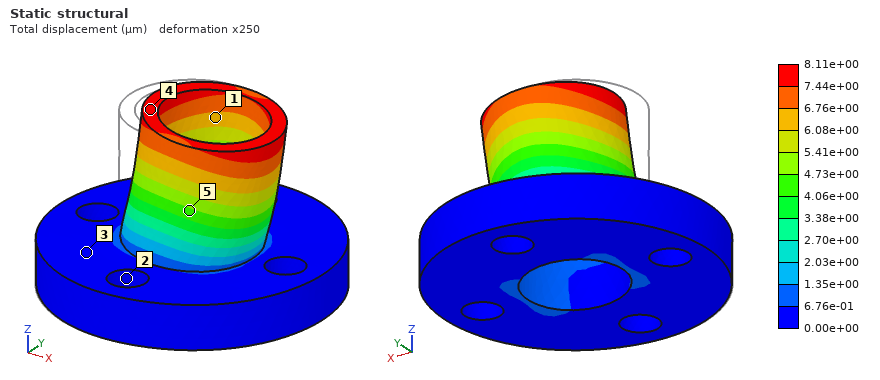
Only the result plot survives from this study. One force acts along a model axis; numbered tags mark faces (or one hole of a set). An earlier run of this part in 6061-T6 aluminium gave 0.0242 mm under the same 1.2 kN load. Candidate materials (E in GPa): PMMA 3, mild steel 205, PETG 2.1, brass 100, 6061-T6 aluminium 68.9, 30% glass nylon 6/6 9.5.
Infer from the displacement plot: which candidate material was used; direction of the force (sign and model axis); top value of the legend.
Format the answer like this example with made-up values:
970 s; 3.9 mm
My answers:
mild steel; +X; 8.11e+00 µm
